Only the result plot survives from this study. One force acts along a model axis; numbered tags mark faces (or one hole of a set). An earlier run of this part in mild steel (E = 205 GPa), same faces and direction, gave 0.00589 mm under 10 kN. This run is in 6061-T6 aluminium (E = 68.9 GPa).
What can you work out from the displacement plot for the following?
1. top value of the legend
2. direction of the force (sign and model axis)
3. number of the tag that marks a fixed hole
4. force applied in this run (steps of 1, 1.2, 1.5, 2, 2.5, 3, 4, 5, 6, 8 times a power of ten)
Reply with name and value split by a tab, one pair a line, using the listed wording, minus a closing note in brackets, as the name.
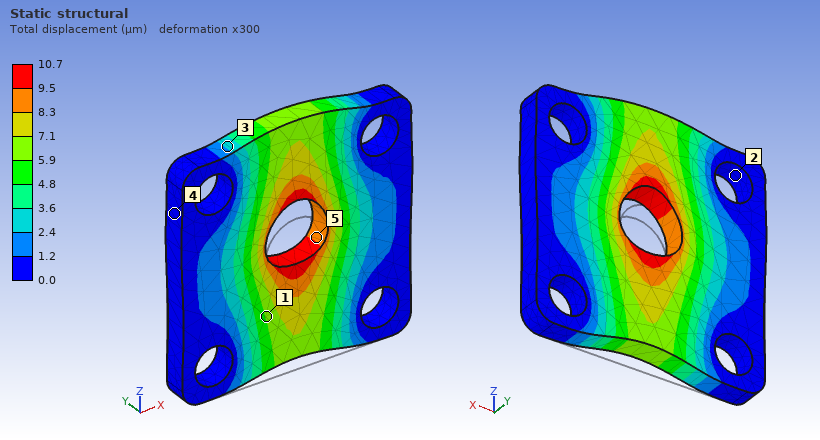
top value of the legend	10.7 µm
direction of the force	+Z
number of the tag that marks a fixed hole	2
force applied in this run	6 kN
